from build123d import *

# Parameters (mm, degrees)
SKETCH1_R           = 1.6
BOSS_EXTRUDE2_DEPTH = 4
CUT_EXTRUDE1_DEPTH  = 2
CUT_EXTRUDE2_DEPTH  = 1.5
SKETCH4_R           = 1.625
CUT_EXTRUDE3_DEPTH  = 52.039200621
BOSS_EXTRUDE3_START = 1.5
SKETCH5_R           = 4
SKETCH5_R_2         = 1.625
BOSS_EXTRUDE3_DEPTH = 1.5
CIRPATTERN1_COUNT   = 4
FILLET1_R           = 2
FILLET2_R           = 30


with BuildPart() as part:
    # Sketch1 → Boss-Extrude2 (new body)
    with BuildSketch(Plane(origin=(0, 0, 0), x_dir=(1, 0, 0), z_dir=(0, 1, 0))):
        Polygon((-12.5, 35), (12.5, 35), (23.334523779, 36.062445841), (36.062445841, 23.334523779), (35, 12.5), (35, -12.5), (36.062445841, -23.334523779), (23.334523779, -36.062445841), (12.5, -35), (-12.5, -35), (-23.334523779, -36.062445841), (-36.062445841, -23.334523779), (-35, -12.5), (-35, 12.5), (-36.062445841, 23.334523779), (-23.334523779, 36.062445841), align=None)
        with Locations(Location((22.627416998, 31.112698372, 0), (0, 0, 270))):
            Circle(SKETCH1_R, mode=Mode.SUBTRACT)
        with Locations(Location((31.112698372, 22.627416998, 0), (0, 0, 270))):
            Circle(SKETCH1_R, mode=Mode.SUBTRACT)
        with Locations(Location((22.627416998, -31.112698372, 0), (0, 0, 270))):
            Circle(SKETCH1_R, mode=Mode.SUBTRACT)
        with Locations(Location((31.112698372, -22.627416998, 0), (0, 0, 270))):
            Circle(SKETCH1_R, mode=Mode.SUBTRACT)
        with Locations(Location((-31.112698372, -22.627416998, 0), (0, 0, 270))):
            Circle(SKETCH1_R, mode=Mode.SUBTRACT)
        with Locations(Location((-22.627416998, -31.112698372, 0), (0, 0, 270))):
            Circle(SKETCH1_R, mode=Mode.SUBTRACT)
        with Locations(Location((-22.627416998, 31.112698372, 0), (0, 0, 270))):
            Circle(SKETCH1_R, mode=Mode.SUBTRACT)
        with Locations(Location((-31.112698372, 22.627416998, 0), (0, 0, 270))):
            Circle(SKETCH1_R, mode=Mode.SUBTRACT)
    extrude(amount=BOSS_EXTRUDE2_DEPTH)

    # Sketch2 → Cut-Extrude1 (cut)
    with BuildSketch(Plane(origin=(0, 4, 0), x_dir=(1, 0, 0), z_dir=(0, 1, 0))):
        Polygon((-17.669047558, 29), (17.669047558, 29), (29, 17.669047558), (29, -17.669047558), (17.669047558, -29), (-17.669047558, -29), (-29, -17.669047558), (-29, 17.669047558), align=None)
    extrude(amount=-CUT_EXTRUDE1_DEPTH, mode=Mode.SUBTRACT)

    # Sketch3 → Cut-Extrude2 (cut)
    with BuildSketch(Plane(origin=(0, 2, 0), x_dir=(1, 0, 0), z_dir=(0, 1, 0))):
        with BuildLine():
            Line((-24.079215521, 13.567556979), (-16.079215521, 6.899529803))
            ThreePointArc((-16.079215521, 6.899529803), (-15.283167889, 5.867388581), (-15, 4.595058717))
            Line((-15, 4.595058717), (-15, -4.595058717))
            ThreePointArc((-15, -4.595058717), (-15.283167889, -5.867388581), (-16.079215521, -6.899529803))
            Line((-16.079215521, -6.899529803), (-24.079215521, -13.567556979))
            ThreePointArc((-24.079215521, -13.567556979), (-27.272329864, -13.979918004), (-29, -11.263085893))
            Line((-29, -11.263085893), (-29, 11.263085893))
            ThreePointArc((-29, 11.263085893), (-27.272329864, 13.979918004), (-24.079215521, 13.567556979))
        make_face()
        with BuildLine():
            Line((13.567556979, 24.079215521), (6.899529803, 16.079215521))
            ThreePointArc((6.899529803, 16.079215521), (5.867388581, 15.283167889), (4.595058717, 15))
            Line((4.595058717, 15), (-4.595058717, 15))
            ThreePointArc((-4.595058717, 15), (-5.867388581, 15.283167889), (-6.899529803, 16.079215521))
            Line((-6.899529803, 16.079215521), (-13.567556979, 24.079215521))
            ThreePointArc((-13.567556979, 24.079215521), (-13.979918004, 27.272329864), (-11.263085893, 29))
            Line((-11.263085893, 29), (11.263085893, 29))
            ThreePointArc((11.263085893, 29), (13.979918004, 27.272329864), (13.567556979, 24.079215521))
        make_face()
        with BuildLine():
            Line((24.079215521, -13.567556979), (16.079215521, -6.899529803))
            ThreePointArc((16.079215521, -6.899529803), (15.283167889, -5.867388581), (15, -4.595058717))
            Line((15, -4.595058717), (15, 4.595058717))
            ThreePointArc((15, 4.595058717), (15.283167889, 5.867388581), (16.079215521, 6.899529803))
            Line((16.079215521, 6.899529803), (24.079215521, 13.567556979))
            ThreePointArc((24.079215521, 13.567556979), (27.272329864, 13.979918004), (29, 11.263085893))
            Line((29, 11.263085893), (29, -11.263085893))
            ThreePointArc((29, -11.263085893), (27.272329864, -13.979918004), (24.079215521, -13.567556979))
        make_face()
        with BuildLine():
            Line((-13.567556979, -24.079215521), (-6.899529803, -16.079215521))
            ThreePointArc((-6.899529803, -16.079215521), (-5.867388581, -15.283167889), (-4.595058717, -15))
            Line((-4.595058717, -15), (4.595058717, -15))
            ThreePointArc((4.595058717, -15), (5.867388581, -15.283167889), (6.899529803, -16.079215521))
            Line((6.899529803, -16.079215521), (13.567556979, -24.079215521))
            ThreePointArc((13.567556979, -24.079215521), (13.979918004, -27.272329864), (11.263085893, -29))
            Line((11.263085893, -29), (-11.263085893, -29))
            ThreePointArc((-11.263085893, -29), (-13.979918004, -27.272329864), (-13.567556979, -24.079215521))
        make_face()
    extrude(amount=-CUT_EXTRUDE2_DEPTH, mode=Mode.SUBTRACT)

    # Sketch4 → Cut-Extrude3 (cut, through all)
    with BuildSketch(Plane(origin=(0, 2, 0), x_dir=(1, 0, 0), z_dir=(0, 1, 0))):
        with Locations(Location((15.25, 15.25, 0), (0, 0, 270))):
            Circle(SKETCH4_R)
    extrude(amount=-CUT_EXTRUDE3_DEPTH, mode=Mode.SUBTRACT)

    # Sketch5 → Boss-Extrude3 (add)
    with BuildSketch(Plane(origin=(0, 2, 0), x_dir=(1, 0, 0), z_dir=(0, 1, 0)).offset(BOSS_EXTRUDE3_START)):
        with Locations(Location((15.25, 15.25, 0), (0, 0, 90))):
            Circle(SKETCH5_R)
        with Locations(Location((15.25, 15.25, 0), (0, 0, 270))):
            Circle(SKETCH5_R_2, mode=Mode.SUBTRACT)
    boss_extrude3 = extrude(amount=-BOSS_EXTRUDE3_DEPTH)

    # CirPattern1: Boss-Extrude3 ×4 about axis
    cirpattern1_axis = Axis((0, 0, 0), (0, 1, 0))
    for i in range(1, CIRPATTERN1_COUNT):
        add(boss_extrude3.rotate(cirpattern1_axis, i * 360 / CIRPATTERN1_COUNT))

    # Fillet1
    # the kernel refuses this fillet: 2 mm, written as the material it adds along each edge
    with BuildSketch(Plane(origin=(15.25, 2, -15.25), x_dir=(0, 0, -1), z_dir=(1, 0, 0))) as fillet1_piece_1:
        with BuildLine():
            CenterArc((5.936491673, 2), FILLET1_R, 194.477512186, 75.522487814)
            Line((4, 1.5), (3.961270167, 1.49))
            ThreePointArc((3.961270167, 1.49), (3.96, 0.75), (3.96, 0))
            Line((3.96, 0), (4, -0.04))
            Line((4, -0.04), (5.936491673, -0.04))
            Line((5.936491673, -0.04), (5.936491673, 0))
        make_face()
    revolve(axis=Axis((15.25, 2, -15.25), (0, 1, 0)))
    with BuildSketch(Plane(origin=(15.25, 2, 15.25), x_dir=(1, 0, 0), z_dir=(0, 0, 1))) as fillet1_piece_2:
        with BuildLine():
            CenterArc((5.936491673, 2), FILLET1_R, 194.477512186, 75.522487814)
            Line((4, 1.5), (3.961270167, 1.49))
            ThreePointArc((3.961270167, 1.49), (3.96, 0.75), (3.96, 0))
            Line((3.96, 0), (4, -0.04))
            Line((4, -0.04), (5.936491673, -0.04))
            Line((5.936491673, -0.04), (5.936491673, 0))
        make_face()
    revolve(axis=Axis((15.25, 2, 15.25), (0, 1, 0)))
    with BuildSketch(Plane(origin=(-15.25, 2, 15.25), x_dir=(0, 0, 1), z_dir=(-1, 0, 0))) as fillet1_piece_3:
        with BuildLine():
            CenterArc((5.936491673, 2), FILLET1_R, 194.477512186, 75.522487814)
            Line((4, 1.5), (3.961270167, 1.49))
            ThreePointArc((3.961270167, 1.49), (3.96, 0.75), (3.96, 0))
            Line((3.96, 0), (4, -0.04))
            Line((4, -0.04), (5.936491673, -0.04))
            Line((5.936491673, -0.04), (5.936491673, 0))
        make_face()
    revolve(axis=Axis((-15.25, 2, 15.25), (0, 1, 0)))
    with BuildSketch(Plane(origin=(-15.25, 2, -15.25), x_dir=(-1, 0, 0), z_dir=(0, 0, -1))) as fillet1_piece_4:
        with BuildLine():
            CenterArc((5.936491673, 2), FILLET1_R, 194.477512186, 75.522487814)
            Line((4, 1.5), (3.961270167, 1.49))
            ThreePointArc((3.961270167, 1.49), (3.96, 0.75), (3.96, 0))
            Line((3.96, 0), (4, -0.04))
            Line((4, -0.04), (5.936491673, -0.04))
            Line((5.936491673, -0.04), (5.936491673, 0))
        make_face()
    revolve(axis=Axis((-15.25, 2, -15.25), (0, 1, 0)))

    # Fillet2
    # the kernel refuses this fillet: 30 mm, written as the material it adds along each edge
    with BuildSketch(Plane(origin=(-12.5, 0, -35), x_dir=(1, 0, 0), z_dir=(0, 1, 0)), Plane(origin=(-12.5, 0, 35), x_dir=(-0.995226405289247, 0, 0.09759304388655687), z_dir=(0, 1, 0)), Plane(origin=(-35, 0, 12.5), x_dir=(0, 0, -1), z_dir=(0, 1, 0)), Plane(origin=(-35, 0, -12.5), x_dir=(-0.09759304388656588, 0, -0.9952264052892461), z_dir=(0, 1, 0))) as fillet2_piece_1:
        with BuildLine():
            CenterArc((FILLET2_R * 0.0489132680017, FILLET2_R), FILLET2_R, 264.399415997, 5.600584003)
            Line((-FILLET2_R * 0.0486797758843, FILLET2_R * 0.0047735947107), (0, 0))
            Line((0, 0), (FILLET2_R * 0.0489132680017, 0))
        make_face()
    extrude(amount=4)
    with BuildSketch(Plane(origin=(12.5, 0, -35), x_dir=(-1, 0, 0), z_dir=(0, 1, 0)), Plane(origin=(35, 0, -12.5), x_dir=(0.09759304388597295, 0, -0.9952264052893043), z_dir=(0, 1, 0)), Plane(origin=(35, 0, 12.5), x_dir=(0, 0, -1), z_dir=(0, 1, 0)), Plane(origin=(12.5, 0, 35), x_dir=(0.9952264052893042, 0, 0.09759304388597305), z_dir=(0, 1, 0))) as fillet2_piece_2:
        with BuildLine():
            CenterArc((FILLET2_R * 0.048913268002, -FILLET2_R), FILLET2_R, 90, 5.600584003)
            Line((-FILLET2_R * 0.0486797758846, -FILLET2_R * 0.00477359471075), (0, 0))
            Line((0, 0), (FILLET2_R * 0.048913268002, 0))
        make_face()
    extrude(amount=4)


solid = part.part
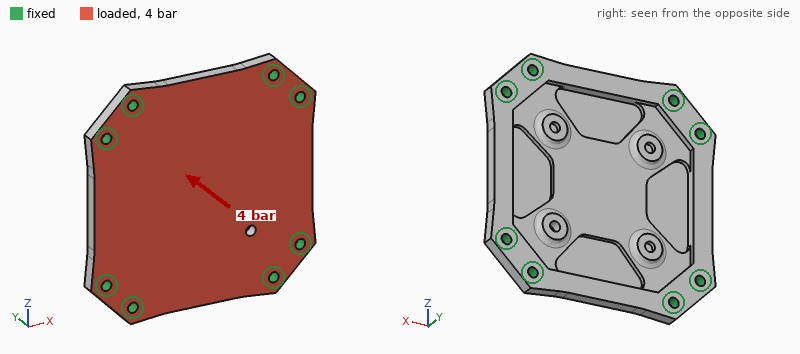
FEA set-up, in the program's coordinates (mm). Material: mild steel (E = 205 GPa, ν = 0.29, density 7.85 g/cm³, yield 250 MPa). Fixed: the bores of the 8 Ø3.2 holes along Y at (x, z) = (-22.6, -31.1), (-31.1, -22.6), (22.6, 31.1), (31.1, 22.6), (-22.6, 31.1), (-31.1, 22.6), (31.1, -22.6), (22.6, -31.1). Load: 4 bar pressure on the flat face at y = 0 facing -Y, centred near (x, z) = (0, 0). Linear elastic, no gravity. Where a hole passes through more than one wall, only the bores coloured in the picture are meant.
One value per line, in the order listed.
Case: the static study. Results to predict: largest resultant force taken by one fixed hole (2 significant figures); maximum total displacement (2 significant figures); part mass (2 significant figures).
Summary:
290 N
0.10 mm
85 g
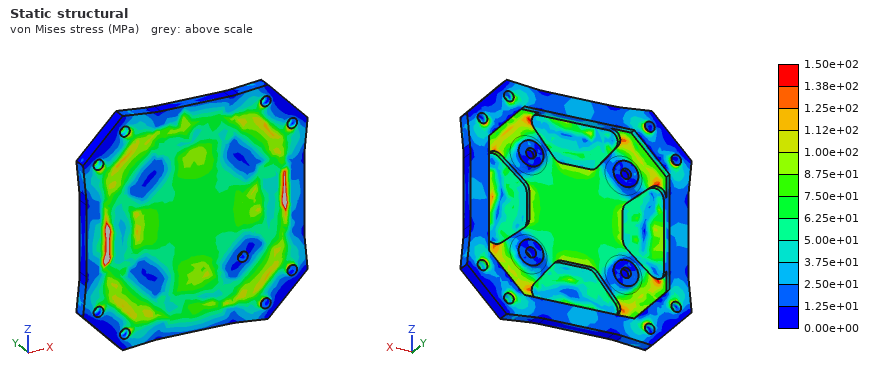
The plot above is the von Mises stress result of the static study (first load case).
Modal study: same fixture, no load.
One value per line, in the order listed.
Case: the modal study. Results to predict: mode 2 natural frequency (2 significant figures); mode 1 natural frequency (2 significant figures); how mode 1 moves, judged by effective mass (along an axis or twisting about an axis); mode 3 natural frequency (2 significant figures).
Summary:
7200 Hz
3300 Hz
along Y
7200 Hz
